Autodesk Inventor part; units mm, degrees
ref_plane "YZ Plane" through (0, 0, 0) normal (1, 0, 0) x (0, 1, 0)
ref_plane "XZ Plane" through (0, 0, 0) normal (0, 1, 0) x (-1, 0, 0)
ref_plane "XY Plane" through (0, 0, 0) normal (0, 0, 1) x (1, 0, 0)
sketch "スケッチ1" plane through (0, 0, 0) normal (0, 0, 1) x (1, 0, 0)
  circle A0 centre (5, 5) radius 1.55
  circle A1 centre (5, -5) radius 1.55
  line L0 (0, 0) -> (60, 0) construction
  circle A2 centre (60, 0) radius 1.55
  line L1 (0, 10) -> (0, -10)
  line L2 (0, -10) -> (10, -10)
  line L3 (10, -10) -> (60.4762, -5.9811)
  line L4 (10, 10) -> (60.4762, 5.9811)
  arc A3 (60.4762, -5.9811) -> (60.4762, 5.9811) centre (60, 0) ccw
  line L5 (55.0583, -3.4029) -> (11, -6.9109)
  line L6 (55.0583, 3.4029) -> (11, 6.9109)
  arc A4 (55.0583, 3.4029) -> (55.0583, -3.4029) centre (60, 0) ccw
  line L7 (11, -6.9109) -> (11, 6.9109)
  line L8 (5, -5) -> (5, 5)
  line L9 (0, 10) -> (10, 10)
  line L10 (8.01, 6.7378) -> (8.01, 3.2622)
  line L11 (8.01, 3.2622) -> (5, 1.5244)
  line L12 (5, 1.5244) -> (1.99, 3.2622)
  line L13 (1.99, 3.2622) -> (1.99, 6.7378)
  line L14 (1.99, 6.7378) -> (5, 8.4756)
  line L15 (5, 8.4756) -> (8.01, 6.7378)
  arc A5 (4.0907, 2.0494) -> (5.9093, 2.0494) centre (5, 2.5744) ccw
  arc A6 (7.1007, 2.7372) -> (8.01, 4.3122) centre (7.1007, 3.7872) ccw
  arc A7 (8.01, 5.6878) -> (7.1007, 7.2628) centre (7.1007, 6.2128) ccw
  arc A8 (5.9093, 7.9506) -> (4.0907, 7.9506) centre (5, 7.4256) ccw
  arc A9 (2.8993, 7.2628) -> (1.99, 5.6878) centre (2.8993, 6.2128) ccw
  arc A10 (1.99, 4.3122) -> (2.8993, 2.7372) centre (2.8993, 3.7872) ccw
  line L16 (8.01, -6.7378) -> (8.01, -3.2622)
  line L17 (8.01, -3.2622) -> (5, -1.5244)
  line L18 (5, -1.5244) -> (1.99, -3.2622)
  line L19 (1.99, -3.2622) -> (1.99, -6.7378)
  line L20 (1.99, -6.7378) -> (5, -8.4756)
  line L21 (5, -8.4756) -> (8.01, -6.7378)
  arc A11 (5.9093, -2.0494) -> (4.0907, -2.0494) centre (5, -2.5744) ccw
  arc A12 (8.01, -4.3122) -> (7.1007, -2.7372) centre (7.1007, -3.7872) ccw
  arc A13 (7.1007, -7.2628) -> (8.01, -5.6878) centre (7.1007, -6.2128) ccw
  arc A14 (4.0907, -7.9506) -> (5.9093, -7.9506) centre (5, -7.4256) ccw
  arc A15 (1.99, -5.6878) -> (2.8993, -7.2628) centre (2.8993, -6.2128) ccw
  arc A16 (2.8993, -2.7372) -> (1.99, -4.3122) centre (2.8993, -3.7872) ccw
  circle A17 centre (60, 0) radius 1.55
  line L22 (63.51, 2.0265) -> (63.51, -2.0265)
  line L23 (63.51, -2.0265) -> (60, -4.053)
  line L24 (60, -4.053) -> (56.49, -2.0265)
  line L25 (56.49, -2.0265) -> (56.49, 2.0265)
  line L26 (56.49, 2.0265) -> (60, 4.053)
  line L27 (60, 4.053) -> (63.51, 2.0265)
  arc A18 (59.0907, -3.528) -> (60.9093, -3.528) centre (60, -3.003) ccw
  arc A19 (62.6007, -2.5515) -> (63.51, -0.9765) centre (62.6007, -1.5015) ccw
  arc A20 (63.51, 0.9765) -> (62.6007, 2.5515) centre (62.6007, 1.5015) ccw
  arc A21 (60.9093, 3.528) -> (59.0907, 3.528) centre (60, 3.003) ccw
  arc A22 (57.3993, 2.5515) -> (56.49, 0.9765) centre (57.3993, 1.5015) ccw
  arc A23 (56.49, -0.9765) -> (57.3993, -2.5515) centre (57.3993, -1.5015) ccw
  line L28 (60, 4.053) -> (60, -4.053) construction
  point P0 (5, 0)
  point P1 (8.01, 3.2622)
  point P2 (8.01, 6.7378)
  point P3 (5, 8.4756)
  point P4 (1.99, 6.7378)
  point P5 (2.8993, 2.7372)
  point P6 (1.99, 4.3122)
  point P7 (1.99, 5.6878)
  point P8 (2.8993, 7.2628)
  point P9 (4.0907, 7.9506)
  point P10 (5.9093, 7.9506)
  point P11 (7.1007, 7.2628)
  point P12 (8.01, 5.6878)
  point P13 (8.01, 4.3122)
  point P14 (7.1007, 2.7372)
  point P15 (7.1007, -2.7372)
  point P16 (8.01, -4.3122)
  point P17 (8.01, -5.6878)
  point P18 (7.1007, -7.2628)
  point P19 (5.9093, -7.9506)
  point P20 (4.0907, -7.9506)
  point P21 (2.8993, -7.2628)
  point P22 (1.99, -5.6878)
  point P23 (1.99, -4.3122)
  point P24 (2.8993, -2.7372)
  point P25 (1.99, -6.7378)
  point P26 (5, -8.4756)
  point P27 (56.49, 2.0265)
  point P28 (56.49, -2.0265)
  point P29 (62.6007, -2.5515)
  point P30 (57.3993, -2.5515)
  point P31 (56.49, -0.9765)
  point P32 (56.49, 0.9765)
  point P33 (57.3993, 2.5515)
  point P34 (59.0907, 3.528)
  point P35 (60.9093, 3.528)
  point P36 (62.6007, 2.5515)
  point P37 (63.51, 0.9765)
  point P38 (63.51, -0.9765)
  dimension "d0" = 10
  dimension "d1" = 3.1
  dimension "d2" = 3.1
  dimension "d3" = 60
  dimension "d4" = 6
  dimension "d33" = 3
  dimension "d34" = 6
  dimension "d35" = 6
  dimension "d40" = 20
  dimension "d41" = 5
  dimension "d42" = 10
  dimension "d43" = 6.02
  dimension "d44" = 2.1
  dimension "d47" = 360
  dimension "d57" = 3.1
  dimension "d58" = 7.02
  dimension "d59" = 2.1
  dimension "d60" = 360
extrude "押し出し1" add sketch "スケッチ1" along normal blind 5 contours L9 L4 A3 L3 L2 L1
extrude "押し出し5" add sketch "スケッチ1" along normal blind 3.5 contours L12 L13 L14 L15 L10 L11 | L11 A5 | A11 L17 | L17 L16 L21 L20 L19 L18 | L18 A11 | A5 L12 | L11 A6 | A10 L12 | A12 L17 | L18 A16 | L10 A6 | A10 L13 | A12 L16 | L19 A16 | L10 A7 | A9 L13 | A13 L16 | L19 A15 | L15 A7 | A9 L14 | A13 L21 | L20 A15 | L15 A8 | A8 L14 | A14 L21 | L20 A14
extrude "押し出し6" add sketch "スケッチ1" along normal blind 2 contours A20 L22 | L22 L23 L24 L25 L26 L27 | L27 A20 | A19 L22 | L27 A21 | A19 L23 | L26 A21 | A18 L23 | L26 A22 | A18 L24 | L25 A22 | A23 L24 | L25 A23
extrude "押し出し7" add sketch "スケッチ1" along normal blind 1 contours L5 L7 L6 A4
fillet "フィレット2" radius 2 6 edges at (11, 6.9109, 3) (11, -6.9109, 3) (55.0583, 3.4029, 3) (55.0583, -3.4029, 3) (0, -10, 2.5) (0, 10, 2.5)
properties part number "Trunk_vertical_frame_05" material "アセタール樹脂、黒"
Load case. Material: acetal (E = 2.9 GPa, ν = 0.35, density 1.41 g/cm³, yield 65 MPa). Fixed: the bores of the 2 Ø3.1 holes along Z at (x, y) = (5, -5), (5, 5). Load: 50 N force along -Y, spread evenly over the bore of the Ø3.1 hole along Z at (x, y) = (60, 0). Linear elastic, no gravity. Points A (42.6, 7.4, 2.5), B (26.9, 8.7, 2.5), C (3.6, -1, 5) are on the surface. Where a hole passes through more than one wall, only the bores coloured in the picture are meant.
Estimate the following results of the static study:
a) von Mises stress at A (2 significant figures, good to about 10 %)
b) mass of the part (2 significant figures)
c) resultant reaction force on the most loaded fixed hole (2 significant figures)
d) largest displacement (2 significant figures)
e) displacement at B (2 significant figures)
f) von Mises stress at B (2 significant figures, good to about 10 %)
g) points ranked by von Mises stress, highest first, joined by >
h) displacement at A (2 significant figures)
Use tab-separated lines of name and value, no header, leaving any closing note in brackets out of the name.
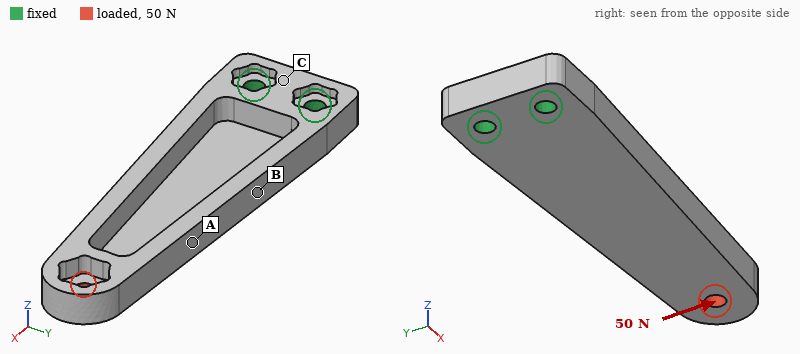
von Mises stress at A	6.1 MPa
mass of the part	4.5 g
resultant reaction force on the most loaded fixed hole	220 N
largest displacement	0.83 mm
displacement at B	0.18 mm
von Mises stress at B	9.1 MPa
points ranked by von Mises stress, highest first, joined by >	B > A > C
displacement at A	0.41 mm
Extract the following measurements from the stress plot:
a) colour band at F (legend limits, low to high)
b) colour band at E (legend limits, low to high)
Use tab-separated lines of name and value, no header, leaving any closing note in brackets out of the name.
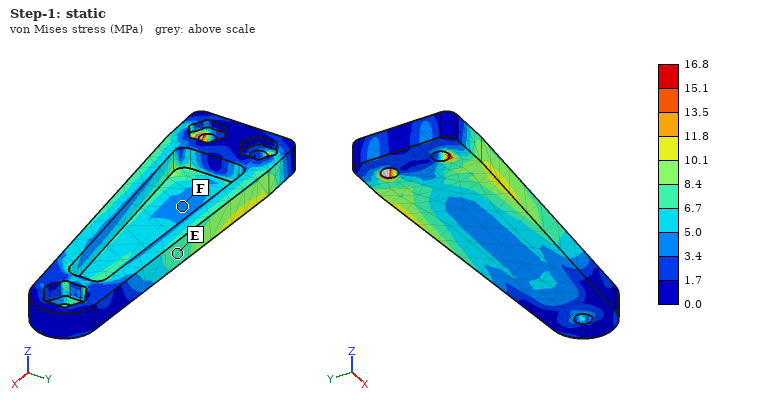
colour band at F	3.4 to 5.0 MPa
colour band at E	6.7 to 8.4 MPa
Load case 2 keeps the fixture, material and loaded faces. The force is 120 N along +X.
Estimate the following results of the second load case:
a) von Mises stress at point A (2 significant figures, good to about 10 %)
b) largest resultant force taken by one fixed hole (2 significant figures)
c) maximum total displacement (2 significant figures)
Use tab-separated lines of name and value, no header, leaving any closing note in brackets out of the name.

von Mises stress at point A	2.5 MPa
largest resultant force taken by one fixed hole	60 N
maximum total displacement	0.72 mm
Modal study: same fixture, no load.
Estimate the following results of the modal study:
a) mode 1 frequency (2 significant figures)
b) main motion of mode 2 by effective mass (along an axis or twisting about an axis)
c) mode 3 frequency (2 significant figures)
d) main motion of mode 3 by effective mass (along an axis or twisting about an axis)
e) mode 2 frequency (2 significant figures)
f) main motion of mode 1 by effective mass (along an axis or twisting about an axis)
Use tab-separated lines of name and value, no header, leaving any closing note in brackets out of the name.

mode 1 frequency	340 Hz
main motion of mode 2 by effective mass	along Y
mode 3 frequency	1500 Hz
main motion of mode 3 by effective mass	along Y
mode 2 frequency	1000 Hz
main motion of mode 1 by effective mass	along Z
